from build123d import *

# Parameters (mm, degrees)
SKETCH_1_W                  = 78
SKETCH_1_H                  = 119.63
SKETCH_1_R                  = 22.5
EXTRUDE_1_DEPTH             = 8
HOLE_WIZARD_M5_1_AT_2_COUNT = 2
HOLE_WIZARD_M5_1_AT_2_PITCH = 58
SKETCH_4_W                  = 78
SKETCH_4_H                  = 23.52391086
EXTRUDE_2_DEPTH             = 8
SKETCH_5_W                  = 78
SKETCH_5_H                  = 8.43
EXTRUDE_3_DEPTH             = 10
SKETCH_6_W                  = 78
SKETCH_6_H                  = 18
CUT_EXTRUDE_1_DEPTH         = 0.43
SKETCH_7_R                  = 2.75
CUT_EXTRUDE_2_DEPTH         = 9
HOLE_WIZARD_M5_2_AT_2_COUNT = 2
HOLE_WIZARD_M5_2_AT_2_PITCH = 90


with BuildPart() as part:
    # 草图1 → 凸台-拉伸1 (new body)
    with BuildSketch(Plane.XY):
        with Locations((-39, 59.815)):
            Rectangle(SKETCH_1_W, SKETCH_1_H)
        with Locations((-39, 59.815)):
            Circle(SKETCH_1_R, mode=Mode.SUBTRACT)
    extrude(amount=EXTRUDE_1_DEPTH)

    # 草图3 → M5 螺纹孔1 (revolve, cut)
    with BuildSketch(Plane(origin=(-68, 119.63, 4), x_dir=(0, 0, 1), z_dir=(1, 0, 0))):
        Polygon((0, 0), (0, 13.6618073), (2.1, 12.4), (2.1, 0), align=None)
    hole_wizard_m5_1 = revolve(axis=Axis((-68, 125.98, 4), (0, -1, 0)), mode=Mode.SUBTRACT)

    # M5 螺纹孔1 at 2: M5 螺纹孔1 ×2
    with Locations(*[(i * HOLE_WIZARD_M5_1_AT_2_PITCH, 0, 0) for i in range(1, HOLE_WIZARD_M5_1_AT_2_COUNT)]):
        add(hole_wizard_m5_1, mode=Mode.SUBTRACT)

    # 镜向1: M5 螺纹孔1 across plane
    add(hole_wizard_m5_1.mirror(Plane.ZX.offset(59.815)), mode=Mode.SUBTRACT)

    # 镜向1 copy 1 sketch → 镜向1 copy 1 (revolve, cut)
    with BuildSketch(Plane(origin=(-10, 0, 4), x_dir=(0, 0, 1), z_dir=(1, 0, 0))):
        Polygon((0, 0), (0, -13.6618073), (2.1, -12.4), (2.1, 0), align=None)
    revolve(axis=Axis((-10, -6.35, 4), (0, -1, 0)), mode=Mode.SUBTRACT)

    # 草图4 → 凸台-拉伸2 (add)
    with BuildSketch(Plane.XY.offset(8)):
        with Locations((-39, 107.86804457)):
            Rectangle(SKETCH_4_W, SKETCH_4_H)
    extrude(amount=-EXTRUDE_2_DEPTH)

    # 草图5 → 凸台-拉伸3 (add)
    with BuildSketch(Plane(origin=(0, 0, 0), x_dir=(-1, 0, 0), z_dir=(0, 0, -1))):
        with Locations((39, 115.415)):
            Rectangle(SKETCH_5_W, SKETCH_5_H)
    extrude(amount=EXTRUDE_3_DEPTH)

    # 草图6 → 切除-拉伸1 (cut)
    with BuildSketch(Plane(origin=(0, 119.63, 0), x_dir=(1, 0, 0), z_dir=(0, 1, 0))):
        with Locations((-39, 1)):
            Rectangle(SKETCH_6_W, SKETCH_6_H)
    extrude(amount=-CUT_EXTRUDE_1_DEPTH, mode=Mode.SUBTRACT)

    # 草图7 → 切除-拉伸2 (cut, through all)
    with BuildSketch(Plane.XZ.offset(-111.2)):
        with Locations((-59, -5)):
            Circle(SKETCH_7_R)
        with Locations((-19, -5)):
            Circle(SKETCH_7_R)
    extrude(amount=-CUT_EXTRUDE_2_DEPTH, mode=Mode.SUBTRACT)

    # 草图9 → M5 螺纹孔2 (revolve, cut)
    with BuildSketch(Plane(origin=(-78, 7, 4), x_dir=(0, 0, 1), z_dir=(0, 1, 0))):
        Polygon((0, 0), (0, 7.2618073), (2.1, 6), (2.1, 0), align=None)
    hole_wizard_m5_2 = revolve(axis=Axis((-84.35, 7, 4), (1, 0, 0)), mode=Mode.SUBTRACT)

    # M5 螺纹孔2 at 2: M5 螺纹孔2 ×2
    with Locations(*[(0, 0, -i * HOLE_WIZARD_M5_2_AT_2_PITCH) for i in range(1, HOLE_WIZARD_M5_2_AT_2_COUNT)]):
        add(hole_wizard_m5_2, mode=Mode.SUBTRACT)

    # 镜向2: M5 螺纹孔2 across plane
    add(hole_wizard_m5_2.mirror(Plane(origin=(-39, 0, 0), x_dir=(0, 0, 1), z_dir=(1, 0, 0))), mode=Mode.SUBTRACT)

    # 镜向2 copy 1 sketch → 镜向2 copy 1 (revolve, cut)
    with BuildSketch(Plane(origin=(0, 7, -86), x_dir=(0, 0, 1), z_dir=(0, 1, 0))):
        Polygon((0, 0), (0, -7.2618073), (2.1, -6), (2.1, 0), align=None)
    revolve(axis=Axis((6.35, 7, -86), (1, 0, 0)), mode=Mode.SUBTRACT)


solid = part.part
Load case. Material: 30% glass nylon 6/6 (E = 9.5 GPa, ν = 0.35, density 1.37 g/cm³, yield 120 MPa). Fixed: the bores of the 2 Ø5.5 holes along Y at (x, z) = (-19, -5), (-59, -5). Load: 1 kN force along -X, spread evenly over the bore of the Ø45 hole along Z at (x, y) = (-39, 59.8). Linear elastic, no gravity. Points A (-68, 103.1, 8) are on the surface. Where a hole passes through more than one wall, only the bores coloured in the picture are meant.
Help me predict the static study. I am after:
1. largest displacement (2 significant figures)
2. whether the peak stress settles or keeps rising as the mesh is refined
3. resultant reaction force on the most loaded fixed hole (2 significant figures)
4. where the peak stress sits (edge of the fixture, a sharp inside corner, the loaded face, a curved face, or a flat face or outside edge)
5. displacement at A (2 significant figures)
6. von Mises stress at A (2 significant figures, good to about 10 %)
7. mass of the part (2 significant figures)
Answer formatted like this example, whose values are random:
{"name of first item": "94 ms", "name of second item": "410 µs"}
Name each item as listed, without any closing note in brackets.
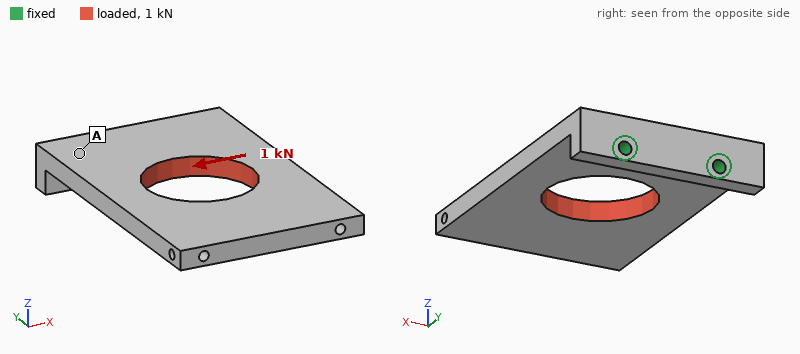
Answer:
{"largest displacement": "0.43 mm", "whether the peak stress settles or keeps rising as the mesh is refined": "keeps rising", "resultant reaction force on the most loaded fixed hole": "1.3 kN", "where the peak stress sits": "edge of the fixture", "displacement at A": "0.088 mm", "von Mises stress at A": "5.8 MPa", "mass of the part": "92 g"}
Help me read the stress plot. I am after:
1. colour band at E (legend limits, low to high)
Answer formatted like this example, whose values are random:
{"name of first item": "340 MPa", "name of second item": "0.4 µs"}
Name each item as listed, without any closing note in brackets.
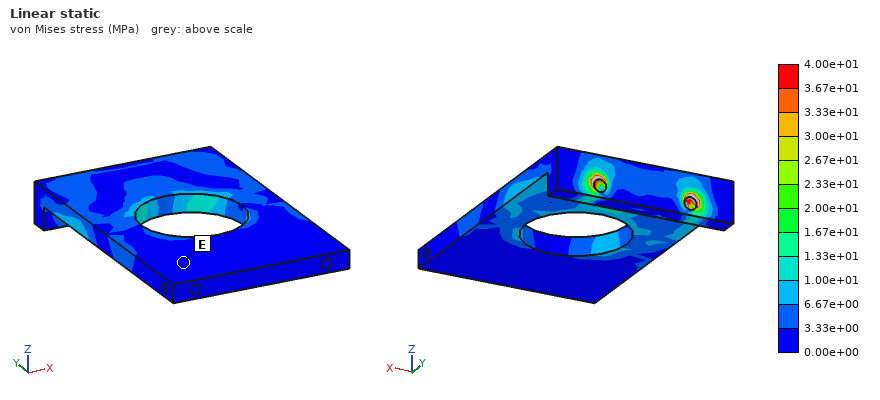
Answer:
{"colour band at E": "0.00e+00 to 3.33e+00 MPa"}
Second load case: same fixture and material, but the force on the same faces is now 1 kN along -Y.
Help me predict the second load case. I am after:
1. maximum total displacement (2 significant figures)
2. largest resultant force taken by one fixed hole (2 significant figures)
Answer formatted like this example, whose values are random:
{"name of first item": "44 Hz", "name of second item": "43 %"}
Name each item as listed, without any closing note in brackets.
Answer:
{"maximum total displacement": "0.28 mm", "largest resultant force taken by one fixed hole": "500 N"}
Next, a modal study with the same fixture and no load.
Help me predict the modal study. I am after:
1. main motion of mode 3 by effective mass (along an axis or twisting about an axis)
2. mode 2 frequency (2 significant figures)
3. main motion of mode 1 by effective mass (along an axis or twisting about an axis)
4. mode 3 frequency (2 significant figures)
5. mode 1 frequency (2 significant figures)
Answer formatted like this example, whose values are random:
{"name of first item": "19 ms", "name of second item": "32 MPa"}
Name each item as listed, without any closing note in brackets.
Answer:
{"main motion of mode 3 by effective mass": "along X", "mode 2 frequency": "680 Hz", "main motion of mode 1 by effective mass": "along Z", "mode 3 frequency": "1000 Hz", "mode 1 frequency": "210 Hz"}
